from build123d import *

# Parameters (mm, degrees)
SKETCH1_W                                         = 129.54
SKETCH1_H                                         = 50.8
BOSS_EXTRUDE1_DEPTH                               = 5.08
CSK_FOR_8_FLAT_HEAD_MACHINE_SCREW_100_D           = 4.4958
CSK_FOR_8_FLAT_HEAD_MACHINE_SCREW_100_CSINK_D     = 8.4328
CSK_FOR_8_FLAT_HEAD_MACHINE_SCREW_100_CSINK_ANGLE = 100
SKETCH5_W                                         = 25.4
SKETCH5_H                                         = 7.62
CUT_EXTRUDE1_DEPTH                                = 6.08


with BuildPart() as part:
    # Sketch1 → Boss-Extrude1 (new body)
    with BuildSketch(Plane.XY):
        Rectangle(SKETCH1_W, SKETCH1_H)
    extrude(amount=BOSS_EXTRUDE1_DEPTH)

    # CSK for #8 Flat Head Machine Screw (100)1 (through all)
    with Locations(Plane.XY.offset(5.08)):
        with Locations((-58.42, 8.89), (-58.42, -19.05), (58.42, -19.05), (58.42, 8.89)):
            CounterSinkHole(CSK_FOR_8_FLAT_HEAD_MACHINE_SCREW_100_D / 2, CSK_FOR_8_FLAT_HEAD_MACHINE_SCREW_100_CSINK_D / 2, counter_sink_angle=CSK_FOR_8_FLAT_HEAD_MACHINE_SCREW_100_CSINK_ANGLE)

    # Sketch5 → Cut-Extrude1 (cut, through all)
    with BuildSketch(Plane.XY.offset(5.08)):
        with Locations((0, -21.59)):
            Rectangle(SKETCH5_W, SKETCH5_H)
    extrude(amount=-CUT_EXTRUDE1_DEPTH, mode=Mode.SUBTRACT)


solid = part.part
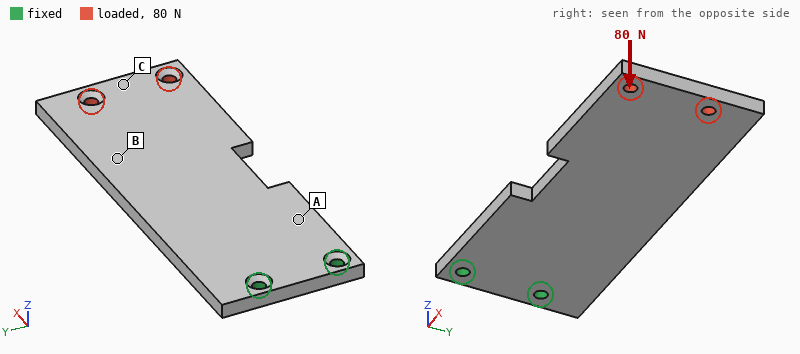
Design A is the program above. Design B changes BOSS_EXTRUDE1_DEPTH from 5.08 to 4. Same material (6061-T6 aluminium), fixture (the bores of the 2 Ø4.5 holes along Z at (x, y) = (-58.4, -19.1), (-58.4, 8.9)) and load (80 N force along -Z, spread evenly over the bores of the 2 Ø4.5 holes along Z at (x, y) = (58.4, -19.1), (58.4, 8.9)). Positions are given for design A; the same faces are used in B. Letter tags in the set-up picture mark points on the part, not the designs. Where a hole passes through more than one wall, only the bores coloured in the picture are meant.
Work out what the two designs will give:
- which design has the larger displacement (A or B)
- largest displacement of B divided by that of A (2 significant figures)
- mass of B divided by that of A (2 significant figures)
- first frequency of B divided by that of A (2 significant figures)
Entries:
B
1.9
0.79
0.82
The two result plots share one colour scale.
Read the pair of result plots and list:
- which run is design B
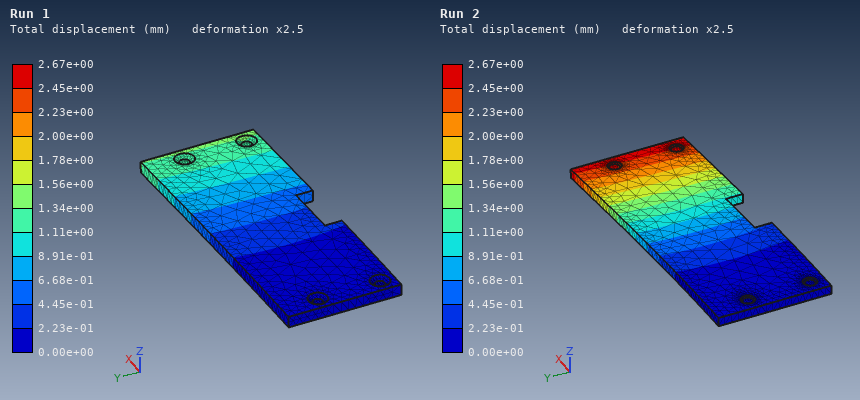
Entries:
Run 2
